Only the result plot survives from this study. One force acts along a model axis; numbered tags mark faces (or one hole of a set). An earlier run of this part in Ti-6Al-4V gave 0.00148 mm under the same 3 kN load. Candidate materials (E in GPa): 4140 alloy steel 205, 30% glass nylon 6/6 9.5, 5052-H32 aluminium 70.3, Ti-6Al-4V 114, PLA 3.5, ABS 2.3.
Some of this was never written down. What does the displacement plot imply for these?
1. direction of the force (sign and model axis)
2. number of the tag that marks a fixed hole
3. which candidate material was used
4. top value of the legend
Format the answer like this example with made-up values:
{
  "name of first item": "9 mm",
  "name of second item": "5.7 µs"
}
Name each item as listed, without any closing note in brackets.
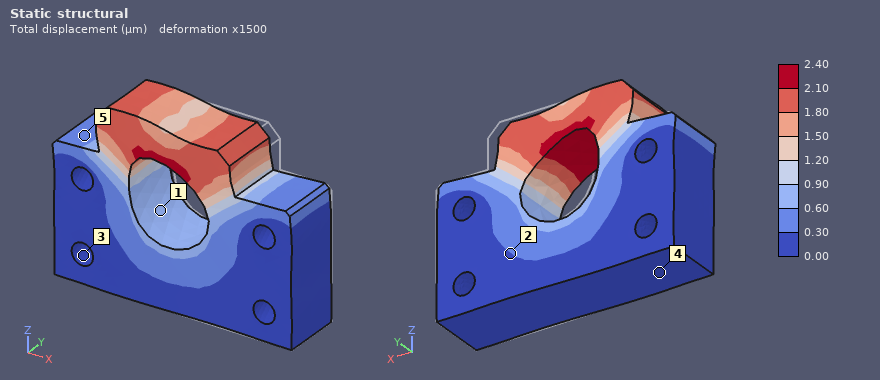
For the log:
{
  "direction of the force": "-X",
  "number of the tag that marks a fixed hole": "3",
  "which candidate material was used": "5052-H32 aluminium",
  "top value of the legend": "2.40 µm"
}
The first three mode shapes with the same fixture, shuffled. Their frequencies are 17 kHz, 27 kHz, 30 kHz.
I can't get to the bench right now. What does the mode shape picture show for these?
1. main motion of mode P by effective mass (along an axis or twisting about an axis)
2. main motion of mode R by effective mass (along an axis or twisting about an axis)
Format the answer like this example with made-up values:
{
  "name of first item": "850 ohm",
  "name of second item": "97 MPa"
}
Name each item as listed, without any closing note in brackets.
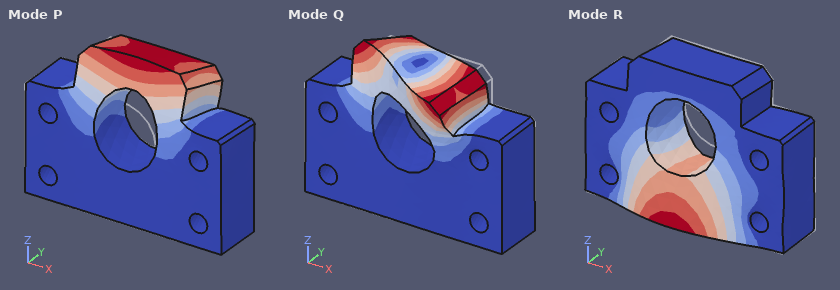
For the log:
{
  "main motion of mode P by effective mass": "along Y",
  "main motion of mode R by effective mass": "along Y"
}
